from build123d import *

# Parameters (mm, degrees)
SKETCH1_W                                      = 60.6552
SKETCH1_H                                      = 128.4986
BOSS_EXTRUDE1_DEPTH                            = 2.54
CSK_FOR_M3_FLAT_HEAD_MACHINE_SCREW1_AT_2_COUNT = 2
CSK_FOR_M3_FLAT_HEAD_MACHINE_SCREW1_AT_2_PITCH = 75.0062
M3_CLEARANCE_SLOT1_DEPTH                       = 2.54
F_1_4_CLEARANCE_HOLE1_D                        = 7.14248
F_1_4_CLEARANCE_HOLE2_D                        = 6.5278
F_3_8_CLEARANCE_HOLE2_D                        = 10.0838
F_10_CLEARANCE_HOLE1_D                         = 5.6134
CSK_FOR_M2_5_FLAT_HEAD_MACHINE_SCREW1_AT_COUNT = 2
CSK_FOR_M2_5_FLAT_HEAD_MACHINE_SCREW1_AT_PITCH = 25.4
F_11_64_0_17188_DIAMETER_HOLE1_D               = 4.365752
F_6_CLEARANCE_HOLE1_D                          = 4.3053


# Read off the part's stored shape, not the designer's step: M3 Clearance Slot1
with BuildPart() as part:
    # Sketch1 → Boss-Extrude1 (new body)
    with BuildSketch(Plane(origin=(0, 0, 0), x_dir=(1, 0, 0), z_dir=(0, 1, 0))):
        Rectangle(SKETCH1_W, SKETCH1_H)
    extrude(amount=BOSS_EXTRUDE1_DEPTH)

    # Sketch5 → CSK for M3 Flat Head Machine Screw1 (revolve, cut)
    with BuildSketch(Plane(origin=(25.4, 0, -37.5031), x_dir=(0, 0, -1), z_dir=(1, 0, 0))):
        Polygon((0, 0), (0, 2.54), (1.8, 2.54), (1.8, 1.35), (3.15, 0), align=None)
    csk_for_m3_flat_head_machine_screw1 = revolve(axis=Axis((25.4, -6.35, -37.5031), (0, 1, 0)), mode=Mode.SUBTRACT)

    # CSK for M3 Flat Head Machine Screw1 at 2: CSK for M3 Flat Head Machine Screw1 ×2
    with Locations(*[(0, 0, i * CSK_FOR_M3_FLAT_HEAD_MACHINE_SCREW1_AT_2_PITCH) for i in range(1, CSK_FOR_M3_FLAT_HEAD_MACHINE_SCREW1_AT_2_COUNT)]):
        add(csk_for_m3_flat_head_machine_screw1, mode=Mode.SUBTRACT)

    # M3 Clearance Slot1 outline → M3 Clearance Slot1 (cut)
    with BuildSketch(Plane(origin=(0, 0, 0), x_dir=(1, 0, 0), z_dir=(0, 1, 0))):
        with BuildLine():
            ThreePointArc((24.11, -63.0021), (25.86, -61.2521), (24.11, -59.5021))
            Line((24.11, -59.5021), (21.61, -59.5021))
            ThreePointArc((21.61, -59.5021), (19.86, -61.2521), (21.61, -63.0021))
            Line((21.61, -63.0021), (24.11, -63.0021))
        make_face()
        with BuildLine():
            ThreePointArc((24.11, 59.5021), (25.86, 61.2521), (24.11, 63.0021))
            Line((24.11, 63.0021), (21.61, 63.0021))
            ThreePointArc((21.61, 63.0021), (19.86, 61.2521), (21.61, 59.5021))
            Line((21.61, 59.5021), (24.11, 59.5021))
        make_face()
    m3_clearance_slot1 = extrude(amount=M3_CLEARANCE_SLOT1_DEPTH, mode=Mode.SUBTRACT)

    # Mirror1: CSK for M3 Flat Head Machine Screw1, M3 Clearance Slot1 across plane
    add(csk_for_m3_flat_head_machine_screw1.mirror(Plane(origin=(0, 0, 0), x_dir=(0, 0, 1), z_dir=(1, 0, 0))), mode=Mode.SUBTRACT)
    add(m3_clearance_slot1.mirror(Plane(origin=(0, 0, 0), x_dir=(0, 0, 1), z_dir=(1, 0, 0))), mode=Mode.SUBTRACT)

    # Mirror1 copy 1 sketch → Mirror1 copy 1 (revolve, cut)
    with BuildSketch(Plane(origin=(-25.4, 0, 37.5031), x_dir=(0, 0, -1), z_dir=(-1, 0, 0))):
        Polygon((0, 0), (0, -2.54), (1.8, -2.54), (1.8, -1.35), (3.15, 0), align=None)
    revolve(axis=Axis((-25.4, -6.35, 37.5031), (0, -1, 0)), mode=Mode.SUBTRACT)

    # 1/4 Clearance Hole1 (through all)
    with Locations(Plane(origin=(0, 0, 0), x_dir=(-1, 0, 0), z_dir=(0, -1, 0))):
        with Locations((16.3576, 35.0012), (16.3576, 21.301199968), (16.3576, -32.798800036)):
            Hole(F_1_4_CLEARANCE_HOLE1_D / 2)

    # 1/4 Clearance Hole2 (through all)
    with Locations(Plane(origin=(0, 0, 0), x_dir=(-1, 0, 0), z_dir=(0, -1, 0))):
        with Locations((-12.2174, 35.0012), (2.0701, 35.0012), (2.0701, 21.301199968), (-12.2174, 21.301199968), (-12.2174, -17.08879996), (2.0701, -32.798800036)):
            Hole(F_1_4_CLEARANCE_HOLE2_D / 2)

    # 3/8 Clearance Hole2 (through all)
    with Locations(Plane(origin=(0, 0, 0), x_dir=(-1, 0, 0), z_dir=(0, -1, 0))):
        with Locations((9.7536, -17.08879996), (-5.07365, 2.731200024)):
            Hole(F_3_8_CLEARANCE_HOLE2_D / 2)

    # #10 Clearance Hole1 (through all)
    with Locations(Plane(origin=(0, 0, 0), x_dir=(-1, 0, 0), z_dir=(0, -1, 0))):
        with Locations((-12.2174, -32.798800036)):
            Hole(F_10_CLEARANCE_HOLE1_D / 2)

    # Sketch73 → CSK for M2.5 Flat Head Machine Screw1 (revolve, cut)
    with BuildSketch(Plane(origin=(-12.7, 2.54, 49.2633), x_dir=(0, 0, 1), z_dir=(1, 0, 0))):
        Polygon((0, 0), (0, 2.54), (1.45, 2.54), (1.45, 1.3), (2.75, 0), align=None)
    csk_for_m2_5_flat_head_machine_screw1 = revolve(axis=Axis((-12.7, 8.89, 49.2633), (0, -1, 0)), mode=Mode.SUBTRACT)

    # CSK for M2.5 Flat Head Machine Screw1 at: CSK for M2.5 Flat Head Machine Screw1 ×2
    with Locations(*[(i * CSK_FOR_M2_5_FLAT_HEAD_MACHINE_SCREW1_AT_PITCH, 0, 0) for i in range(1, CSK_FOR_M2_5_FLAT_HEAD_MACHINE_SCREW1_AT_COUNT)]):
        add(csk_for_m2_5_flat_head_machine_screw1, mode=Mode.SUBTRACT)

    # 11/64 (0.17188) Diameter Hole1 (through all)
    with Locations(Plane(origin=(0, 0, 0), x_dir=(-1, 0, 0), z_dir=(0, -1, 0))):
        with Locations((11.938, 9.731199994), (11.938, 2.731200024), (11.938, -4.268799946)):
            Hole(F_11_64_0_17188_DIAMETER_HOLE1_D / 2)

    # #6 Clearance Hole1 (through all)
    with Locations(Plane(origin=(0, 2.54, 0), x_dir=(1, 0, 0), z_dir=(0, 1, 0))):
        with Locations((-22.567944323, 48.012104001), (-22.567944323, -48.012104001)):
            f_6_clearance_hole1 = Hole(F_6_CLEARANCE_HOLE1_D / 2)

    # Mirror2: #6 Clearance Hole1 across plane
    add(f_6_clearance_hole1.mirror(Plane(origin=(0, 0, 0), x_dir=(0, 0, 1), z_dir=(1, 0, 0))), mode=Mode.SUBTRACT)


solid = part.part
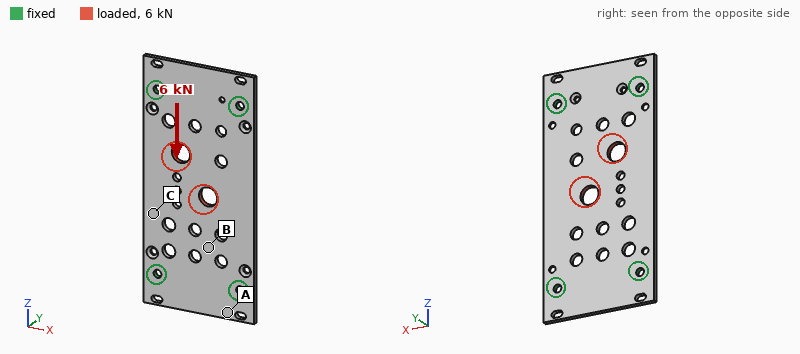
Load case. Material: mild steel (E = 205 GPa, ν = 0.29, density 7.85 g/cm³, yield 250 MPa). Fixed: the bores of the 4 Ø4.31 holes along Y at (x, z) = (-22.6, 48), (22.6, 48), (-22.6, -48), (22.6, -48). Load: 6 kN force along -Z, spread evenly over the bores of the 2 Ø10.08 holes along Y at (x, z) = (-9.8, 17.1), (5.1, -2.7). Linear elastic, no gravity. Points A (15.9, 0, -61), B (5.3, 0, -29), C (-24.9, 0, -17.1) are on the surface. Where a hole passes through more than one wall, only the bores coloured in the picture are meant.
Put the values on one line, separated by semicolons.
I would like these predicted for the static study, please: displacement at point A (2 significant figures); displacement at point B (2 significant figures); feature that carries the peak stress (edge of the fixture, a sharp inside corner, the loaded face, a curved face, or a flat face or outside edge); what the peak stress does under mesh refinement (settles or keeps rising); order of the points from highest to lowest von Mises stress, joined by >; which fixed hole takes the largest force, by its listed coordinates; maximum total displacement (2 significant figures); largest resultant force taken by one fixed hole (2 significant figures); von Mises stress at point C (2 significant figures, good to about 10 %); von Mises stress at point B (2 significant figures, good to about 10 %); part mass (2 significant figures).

1.5 µm; 4.2 µm; a sharp inside corner; keeps rising; B > C > A; (-22.6, 48); 9.5 µm; 1.8 kN; 16 MPa; 32 MPa; 140 g
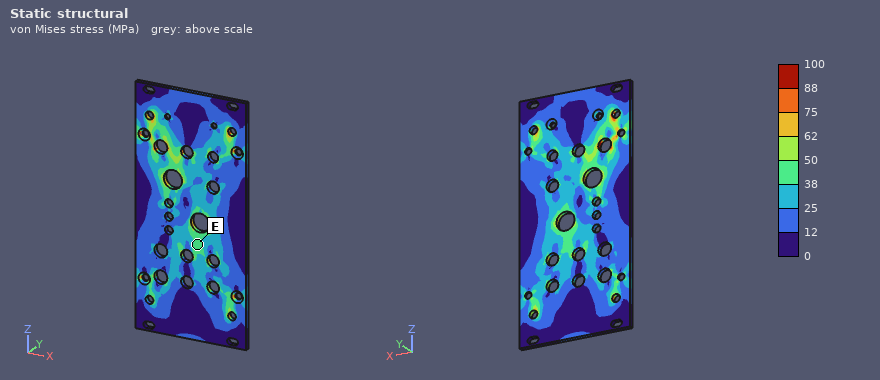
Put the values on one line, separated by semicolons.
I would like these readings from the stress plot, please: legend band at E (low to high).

38 to 50 MPa
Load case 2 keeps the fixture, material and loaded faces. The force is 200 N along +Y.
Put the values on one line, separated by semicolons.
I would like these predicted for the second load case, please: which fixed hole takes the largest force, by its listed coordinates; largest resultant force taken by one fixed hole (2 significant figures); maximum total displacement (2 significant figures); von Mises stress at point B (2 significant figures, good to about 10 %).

(-22.6, 48); 73 N; 68 µm; 10 MPa
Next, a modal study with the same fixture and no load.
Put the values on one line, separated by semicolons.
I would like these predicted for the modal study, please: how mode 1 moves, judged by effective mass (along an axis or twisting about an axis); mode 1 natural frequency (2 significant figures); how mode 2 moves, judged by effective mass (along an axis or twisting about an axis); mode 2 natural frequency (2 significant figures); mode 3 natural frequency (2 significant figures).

along Y; 1300 Hz; twisting about Z; 2000 Hz; 3600 Hz
